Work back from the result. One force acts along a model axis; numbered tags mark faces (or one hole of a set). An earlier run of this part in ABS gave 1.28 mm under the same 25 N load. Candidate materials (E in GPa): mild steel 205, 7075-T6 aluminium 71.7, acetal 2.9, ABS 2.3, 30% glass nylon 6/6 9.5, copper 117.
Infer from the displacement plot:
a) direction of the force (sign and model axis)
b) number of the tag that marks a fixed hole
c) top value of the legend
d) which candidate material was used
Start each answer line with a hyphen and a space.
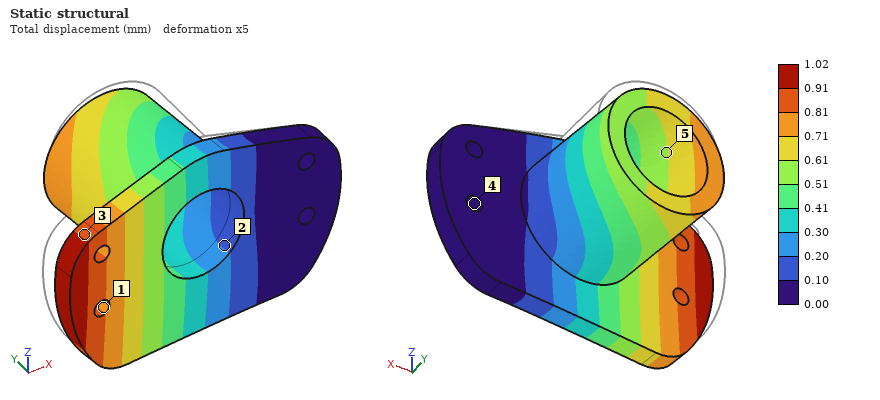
- -Y
- 4
- 1.02 mm
- acetal
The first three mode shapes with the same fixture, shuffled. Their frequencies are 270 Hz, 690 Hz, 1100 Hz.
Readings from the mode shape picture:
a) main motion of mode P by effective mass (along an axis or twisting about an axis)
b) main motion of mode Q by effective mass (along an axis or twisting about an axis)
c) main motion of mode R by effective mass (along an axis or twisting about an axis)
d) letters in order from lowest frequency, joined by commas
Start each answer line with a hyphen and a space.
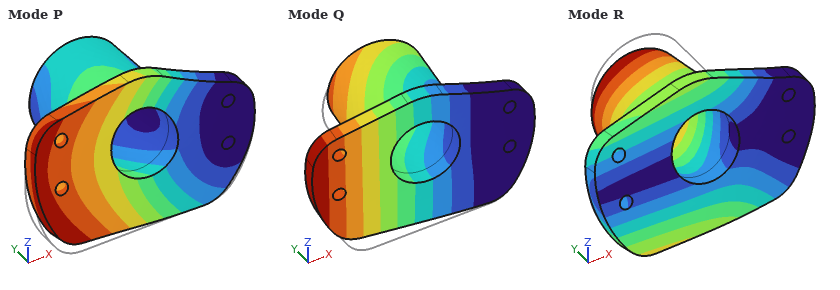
- along Z
- along Y
- along Z
- Q, R, P
